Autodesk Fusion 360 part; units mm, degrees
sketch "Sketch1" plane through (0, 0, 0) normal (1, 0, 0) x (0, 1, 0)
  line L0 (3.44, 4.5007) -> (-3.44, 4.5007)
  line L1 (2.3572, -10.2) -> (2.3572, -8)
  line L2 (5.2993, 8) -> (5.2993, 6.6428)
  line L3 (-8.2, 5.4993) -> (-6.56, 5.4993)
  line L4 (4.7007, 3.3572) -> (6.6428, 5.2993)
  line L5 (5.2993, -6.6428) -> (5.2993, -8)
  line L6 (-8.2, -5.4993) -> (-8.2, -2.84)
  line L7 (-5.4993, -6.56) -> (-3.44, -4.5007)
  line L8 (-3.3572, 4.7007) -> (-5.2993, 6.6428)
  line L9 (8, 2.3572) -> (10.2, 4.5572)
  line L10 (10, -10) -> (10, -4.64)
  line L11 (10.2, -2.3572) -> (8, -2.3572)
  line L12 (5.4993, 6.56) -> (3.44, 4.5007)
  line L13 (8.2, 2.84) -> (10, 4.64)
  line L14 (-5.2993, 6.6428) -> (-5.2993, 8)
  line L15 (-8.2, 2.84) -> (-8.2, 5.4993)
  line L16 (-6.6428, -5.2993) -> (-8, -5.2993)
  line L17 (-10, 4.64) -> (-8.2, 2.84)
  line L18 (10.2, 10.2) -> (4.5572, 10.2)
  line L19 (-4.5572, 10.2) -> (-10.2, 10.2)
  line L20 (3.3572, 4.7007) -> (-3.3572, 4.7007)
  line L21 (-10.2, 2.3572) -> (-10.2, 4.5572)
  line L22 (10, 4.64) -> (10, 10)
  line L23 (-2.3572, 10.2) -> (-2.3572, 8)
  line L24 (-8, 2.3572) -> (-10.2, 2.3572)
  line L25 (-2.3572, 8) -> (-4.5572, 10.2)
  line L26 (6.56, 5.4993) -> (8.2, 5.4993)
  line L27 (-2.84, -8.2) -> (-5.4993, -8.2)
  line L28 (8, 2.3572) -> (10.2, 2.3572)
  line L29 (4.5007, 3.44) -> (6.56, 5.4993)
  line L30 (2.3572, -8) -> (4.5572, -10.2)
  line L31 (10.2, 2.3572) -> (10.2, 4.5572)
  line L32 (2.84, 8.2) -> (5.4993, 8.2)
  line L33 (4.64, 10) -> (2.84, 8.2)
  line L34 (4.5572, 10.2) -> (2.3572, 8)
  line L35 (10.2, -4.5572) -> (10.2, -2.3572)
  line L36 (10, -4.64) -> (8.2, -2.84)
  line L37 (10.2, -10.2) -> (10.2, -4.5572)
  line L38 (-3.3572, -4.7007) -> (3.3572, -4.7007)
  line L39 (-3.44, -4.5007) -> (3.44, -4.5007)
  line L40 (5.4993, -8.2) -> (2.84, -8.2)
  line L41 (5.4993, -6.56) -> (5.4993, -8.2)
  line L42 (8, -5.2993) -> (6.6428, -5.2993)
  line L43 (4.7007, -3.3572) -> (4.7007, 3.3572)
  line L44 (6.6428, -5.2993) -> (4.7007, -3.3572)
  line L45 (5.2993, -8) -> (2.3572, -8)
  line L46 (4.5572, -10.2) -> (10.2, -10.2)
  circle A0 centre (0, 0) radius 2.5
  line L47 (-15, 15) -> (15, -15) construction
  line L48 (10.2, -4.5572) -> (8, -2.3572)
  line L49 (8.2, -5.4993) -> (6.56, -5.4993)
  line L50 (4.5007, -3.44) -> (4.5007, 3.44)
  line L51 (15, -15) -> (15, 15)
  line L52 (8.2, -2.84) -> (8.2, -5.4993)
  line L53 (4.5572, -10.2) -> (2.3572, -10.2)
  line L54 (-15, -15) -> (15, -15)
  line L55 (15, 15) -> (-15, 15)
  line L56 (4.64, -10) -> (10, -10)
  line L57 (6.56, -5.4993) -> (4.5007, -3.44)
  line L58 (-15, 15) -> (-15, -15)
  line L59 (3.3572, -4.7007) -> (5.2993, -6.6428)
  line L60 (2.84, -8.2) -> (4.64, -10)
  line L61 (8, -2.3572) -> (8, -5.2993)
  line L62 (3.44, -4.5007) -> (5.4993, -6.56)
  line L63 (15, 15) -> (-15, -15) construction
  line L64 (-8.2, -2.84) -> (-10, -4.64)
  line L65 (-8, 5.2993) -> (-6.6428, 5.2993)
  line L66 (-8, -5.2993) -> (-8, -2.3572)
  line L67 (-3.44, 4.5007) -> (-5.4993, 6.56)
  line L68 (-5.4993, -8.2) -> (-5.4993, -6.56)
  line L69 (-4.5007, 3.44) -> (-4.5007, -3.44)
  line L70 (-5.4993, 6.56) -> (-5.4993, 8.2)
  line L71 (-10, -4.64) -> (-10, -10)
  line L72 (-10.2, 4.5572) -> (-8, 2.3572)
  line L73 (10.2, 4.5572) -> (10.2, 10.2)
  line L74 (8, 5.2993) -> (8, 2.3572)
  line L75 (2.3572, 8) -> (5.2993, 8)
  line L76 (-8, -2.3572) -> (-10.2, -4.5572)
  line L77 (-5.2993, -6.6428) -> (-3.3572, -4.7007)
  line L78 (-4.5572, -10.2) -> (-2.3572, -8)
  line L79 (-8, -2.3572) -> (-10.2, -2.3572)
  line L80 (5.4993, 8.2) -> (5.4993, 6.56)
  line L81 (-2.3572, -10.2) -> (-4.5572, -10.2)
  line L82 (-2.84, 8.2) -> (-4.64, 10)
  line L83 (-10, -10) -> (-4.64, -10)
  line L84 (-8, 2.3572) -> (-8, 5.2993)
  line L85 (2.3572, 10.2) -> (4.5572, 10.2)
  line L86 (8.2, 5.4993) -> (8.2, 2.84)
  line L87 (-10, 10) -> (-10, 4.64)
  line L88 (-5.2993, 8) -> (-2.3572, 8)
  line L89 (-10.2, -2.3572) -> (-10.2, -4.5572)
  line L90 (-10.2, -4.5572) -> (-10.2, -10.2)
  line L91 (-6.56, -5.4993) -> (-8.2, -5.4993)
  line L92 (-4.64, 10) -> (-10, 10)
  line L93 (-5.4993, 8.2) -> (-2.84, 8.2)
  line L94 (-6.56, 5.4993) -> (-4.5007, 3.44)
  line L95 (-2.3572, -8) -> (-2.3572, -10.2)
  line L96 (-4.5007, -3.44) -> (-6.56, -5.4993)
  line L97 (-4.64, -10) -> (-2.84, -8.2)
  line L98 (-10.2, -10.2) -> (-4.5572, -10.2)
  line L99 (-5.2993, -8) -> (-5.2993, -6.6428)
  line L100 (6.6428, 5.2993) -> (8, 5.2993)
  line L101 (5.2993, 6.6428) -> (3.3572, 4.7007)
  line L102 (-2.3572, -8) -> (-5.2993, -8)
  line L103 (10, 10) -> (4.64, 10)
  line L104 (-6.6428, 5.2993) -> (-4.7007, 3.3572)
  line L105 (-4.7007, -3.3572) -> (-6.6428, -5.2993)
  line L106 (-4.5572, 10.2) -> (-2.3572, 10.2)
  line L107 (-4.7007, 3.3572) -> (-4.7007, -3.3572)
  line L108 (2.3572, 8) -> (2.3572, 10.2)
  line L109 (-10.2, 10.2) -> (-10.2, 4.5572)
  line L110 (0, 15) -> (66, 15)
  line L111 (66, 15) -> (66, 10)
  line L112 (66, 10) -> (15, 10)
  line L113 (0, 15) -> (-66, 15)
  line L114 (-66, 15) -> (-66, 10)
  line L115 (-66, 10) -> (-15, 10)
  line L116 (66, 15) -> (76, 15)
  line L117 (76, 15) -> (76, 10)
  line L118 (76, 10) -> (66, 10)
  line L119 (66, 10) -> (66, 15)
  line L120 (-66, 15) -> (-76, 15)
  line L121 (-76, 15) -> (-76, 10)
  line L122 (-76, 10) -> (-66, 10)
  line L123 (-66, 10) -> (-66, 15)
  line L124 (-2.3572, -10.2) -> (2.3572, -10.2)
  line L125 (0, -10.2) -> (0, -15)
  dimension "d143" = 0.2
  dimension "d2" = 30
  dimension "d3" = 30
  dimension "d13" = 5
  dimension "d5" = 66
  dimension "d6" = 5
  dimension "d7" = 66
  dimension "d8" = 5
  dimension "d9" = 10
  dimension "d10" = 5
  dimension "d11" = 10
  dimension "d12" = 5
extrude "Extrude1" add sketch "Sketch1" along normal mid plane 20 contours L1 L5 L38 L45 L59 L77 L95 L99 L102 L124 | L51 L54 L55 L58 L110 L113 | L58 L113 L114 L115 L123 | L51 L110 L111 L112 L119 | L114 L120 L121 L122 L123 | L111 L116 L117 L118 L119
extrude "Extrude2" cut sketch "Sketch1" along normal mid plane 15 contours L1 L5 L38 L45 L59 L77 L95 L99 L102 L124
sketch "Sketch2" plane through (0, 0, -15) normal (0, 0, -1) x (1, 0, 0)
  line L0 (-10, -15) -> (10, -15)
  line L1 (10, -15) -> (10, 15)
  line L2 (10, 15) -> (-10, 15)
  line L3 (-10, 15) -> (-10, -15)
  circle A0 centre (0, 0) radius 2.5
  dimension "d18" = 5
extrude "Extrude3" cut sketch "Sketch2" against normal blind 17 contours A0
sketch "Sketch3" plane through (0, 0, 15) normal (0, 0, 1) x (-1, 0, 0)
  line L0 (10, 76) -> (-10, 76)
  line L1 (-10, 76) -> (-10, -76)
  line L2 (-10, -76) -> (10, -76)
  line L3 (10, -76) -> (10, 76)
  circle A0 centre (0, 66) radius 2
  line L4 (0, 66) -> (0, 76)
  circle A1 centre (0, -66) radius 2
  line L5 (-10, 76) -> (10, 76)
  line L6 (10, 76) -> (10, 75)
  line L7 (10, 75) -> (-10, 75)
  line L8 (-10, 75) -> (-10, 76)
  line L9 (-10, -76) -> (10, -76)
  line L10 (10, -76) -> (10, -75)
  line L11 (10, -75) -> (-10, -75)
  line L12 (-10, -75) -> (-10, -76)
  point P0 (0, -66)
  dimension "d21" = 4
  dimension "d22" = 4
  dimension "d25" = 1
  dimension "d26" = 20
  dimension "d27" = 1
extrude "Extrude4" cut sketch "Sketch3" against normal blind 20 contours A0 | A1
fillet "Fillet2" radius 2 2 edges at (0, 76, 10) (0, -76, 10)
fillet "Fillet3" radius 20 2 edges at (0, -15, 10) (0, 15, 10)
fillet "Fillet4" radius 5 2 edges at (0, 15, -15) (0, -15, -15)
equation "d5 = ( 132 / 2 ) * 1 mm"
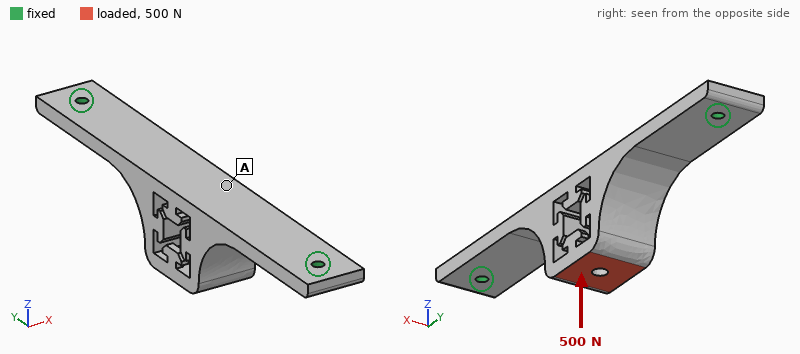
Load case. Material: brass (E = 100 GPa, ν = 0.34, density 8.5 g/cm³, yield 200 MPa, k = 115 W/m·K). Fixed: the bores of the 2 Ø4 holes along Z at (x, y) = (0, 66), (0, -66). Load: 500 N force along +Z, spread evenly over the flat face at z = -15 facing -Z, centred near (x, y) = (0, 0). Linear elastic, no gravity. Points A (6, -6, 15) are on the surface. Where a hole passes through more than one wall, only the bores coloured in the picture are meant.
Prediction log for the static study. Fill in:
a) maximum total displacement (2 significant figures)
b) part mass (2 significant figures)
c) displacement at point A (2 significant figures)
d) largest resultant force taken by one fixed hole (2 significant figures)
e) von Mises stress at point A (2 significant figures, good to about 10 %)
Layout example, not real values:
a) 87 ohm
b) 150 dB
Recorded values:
a) 79 µm
b) 230 g
c) 79 µm
d) 370 N
e) 6.8 MPa
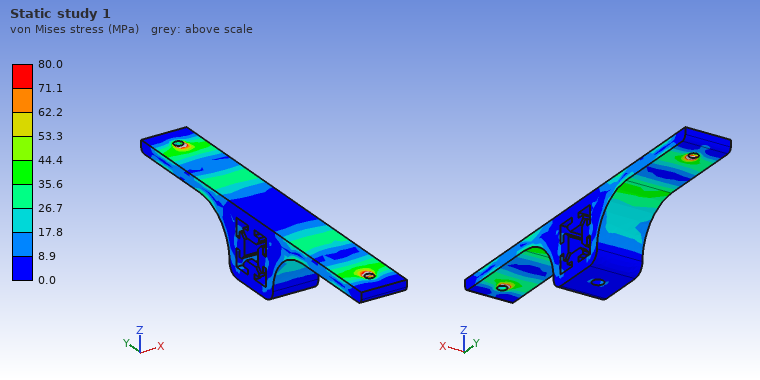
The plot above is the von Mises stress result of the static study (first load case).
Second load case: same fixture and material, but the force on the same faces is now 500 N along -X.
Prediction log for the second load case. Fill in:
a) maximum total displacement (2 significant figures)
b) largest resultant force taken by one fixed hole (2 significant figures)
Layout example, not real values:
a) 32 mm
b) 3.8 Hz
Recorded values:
a) 0.32 mm
b) 250 N
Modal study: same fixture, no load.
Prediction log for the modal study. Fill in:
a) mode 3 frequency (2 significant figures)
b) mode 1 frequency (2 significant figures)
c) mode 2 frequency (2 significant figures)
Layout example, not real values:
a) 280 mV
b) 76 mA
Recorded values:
a) 2300 Hz
b) 970 Hz
c) 970 Hz
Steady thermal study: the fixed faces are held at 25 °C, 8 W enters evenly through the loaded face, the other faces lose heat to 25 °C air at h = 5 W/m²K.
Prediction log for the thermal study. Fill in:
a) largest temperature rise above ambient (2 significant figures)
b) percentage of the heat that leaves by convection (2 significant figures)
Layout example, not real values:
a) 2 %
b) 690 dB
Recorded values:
a) 22 K
b) 9.0 %
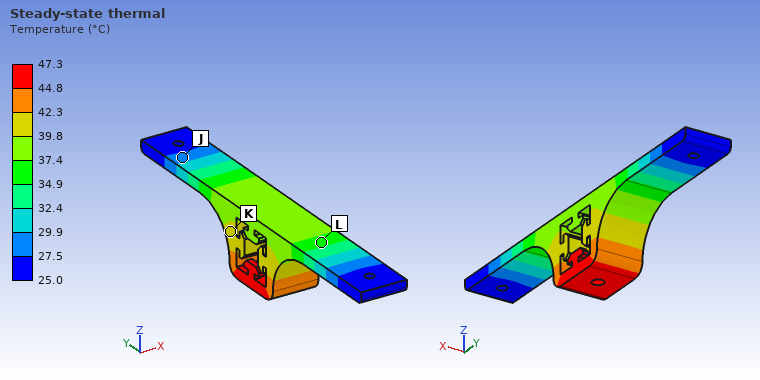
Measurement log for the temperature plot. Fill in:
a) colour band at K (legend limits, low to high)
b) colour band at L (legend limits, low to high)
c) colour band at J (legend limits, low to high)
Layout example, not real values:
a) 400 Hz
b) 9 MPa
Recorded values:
a) 39.8 to 42.3 °C
b) 34.9 to 37.4 °C
c) 27.5 to 29.9 °C
